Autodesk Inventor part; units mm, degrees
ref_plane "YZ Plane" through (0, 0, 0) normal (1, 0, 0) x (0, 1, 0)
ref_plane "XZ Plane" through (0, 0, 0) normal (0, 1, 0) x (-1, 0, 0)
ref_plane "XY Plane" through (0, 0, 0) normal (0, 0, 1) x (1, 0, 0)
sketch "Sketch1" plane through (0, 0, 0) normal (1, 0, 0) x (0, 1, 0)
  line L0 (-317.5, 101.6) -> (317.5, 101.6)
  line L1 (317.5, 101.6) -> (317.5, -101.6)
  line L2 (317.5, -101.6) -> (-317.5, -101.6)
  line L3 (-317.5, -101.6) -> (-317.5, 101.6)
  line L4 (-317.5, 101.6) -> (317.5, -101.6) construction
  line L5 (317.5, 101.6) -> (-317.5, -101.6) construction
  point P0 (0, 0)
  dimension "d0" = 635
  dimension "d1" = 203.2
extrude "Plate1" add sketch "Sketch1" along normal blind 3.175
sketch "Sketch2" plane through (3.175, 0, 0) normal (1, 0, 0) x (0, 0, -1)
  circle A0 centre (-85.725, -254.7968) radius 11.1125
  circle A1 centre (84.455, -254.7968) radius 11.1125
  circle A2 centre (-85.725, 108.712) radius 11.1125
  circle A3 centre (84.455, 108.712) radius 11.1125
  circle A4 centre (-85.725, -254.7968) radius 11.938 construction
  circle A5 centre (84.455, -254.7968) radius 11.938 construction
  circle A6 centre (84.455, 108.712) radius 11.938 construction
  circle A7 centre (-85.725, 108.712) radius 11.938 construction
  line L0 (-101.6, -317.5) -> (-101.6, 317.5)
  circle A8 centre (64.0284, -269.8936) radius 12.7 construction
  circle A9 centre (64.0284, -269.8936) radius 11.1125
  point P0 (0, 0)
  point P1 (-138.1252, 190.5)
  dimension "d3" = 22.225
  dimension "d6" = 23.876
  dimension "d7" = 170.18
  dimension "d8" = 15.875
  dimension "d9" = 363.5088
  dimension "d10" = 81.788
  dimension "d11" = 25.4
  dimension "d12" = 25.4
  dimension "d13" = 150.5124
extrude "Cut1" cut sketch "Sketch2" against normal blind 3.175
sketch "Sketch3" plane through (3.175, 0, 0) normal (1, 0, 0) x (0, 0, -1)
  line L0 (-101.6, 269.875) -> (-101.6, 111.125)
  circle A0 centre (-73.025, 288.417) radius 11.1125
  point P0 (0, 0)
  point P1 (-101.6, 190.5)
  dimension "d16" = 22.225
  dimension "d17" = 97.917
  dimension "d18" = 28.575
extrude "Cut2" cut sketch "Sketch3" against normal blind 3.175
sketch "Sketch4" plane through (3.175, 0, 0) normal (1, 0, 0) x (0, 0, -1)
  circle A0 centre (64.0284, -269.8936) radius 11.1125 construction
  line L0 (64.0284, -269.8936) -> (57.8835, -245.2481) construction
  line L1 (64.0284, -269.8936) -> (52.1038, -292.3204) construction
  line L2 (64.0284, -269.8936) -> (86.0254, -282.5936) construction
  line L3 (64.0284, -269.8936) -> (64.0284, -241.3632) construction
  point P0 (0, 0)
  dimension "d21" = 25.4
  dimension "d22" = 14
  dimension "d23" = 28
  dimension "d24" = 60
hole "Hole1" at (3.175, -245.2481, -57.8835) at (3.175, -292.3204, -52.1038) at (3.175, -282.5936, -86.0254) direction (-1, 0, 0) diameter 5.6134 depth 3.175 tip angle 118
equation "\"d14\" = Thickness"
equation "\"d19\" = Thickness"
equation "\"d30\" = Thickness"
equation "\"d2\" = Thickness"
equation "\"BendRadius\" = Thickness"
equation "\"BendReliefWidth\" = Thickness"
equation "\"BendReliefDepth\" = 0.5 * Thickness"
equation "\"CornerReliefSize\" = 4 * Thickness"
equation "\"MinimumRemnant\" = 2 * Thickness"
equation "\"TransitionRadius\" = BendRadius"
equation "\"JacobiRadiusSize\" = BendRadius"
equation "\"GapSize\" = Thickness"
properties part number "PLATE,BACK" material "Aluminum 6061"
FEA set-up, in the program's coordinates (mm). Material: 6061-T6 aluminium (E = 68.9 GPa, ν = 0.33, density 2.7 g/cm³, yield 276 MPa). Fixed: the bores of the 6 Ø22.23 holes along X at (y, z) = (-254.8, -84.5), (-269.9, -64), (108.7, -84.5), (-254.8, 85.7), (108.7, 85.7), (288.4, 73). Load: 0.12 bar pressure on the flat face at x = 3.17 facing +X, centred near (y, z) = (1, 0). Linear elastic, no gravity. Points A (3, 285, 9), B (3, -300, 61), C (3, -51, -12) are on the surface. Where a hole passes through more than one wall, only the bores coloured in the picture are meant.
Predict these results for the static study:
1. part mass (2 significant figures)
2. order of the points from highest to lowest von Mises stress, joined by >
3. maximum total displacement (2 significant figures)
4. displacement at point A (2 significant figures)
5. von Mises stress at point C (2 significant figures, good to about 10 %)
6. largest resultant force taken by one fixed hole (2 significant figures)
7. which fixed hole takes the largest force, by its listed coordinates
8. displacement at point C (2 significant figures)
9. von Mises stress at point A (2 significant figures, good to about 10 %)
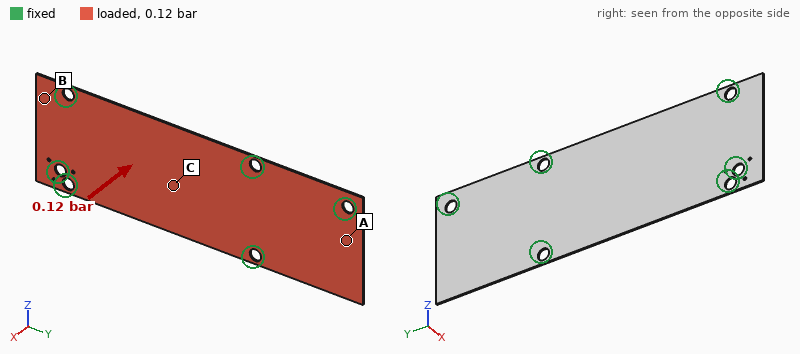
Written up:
1.1 kg
C > A > B
2.9 mm
0.61 mm
32 MPa
410 N
(108.7, -84.5)
2.7 mm
17 MPa
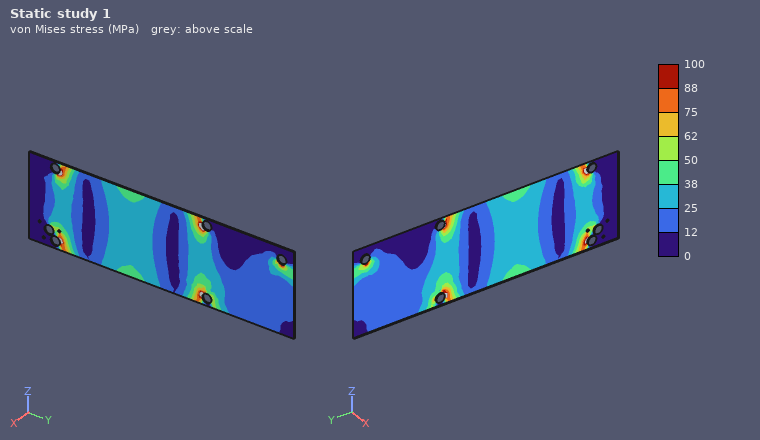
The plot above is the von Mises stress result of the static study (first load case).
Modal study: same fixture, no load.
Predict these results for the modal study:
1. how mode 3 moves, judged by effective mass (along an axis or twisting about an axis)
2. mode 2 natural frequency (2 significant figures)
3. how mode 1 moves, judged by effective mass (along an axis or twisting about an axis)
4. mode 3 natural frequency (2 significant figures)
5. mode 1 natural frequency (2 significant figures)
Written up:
twisting about Y
160 Hz
along X
210 Hz
130 Hz
